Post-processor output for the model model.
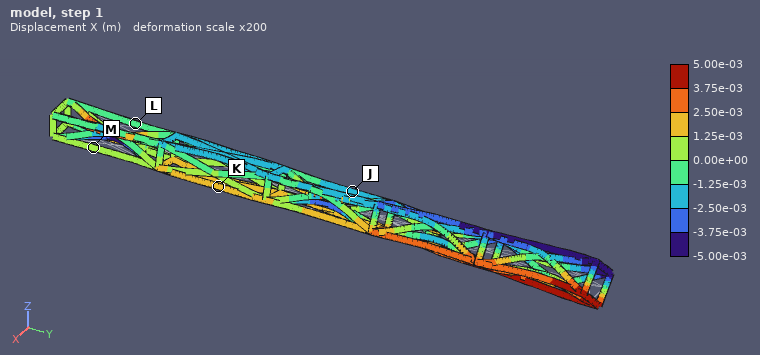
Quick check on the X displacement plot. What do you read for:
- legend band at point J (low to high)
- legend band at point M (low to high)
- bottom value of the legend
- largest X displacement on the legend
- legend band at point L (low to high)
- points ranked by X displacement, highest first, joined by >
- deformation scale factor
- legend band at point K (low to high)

-2.50e-03 to -1.25e-03 m
0.00e+00 to 1.25e-03 m
-5.00e-03 m
5.00e-03 m
-1.25e-03 to 0.00e+00 m
K > M > L > J
200
1.25e-03 to 2.50e-03 m
